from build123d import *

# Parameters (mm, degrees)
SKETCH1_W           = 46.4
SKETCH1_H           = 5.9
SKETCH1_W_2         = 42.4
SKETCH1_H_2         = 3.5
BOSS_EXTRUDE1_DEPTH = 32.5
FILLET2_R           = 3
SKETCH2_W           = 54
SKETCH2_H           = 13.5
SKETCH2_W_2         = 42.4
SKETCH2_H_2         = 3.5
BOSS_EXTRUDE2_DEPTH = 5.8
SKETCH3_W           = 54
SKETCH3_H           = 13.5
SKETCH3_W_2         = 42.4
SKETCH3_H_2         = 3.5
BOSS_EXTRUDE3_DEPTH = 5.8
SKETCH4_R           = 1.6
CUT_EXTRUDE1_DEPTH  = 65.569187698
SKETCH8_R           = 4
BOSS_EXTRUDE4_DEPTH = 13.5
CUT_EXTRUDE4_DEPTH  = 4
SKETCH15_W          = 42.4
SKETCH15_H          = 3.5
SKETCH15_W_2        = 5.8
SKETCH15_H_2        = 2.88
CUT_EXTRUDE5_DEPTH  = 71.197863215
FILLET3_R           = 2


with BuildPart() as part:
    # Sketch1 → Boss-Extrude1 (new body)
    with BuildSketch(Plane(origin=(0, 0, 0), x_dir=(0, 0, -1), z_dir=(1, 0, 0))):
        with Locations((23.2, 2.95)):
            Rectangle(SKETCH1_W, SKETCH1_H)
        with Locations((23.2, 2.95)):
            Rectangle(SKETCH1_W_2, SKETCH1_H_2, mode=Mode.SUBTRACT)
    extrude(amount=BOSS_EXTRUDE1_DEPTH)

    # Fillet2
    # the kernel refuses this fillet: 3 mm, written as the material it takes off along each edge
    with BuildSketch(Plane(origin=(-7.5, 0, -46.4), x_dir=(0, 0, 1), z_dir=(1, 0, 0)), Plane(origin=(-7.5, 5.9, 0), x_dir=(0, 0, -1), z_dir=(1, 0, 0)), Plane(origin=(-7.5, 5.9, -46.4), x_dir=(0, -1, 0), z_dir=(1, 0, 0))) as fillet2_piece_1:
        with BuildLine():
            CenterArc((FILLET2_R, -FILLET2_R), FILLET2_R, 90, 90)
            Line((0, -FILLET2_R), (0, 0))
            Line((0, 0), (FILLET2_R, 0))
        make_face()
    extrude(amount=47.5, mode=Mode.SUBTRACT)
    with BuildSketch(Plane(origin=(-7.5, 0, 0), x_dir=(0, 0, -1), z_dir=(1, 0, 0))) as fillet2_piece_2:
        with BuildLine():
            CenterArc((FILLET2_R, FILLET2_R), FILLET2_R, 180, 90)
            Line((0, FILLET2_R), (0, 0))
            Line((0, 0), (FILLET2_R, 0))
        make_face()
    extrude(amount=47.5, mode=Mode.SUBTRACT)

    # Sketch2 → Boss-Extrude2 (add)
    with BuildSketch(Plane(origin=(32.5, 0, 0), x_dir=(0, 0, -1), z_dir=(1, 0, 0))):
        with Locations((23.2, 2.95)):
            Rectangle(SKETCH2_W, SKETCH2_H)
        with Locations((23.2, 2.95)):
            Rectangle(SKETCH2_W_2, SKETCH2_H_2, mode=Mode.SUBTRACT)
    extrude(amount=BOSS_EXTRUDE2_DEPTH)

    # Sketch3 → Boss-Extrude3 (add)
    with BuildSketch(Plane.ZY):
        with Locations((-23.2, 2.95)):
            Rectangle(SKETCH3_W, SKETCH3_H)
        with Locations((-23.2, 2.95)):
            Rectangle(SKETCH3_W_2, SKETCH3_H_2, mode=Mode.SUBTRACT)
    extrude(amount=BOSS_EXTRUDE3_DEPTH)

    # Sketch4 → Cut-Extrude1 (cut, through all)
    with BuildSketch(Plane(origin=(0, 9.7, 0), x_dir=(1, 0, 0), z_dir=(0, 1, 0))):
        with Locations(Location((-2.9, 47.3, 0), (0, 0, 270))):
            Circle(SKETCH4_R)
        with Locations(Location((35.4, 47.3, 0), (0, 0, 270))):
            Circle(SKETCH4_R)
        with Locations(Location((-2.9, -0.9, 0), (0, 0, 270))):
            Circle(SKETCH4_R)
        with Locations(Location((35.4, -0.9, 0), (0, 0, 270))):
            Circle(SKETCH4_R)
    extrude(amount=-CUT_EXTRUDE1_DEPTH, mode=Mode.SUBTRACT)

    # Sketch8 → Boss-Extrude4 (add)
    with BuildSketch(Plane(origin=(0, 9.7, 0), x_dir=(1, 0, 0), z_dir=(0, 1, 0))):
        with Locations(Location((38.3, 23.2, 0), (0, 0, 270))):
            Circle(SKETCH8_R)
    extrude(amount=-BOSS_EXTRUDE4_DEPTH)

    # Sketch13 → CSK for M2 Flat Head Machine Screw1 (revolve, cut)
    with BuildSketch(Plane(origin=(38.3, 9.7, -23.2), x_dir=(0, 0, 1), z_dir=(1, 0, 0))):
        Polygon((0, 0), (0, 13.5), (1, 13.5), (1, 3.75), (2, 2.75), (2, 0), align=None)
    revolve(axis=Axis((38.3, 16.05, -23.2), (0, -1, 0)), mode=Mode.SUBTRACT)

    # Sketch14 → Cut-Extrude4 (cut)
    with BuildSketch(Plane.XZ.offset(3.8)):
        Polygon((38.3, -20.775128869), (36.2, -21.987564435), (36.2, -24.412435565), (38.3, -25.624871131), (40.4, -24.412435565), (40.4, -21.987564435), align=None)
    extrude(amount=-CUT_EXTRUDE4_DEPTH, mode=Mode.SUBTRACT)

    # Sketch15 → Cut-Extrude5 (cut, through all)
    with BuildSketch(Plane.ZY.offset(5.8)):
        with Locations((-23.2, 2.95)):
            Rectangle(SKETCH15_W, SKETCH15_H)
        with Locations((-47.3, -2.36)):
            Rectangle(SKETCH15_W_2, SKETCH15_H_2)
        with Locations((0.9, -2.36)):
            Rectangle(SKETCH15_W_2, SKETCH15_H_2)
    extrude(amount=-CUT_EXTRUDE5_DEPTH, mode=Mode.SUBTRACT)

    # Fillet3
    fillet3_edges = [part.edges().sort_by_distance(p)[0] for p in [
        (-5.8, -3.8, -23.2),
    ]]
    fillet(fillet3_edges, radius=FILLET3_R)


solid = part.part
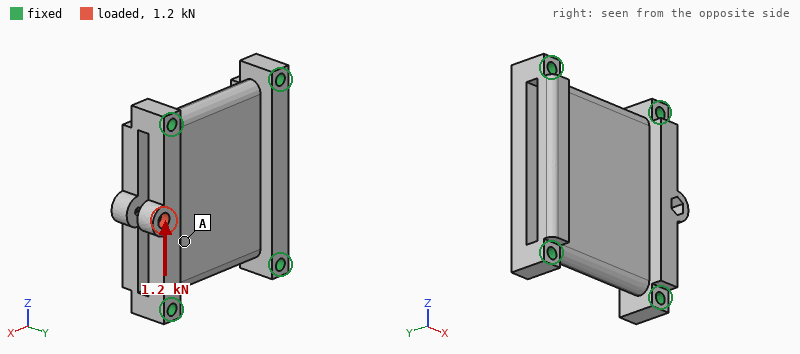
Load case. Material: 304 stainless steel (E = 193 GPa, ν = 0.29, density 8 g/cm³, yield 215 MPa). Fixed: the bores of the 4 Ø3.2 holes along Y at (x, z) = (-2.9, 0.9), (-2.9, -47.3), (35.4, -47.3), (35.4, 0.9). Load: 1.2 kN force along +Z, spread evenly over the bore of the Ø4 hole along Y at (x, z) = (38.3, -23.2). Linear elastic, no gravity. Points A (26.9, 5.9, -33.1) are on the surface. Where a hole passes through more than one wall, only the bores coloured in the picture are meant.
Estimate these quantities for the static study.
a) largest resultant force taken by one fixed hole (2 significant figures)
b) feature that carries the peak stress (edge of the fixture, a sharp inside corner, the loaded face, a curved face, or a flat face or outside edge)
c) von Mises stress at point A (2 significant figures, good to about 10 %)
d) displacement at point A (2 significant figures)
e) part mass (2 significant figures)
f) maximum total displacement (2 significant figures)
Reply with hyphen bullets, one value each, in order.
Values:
- 580 N
- a flat face or outside edge
- 8.7 MPa
- 1.3 µm
- 79 g
- 6.0 µm
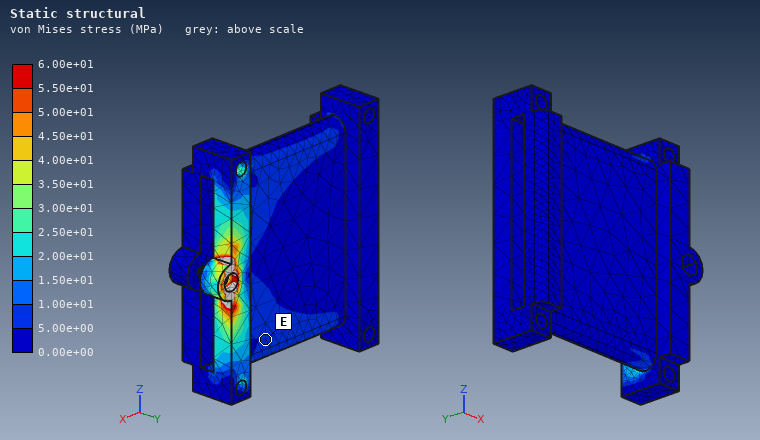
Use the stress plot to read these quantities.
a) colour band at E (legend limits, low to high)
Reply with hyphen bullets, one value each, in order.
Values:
- 5.00e+00 to 1.00e+01 MPa
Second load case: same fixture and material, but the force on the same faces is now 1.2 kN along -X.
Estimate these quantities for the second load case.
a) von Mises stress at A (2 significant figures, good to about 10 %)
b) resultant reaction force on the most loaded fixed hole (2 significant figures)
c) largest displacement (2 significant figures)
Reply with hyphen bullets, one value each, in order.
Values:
- 47 MPa
- 380 N
- 29 µm
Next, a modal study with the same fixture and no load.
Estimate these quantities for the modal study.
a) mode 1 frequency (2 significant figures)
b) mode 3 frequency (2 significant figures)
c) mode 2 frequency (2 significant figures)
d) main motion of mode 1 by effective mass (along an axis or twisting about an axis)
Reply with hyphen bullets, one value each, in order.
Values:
- 5500 Hz
- 7700 Hz
- 6100 Hz
- along Y
